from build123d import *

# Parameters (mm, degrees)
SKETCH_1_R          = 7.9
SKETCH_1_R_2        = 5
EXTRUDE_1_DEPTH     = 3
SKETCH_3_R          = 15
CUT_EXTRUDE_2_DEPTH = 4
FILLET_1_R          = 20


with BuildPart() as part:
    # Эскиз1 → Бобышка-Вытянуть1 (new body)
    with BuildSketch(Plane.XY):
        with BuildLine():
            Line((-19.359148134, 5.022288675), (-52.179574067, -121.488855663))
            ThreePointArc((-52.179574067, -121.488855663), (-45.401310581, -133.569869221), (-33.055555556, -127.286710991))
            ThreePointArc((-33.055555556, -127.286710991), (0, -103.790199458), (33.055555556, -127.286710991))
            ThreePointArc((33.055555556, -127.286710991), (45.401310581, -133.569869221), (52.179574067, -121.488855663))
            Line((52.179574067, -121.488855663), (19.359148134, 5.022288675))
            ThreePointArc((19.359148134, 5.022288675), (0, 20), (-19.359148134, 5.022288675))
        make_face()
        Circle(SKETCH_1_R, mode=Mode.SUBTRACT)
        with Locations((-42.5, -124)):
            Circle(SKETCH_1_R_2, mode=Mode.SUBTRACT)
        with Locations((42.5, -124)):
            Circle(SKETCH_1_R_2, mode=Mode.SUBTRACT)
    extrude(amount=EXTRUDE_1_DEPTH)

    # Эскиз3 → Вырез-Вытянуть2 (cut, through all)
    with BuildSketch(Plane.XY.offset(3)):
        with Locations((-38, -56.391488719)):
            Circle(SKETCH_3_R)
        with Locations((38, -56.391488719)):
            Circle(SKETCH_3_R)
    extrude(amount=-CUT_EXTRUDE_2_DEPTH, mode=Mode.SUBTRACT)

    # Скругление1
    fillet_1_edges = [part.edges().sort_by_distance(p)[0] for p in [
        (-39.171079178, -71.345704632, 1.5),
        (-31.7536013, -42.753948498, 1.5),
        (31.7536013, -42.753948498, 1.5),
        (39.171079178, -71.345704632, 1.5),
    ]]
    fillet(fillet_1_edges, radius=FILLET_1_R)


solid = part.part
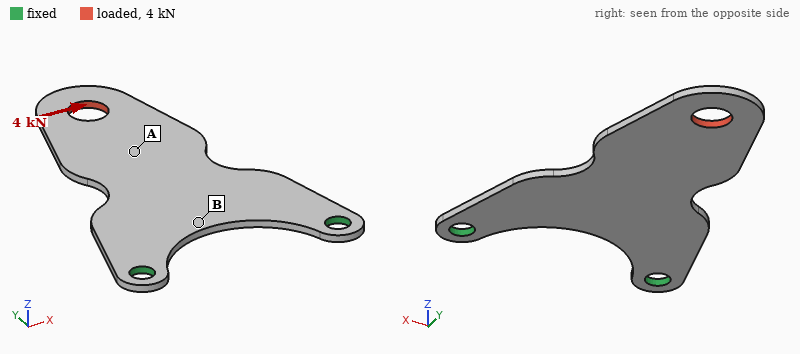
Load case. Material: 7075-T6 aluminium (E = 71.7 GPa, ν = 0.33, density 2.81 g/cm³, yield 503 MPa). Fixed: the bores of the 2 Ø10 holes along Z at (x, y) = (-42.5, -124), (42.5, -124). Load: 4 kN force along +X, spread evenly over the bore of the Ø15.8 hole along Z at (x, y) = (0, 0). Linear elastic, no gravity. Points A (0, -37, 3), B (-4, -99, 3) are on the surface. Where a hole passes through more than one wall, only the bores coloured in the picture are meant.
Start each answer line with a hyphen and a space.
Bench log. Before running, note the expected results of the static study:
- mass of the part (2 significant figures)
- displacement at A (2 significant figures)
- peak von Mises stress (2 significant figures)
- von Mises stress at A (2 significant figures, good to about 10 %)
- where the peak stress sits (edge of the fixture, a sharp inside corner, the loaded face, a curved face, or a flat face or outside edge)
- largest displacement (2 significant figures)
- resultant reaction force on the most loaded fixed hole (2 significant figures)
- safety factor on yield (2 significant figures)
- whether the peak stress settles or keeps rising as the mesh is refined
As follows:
- 69 g
- 0.23 mm
- 340 MPa
- 78 MPa
- a curved face
- 0.68 mm
- 6.1 kN
- 1.5
- settles
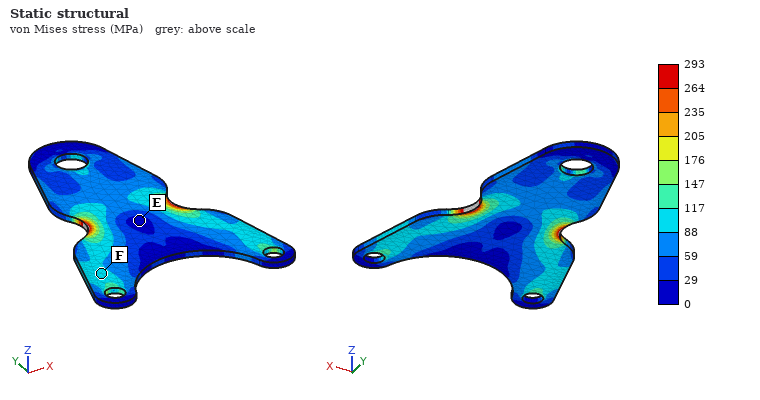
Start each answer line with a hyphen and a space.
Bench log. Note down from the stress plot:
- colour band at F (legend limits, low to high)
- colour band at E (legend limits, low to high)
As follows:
- 88 to 117 MPa
- 0 to 29 MPa
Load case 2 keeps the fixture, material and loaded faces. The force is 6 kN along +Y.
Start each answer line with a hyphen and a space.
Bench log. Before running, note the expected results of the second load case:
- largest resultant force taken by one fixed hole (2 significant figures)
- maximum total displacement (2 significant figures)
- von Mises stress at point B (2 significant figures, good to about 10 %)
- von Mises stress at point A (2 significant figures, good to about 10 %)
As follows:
- 3.3 kN
- 96 µm
- 9.2 MPa
- 43 MPa
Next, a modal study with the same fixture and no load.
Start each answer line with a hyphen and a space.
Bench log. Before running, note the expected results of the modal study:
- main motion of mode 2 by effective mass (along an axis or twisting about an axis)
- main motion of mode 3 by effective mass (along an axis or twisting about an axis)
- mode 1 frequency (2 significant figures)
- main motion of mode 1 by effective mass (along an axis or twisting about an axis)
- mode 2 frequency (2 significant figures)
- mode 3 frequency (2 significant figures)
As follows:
- along Z
- twisting about Y
- 150 Hz
- along Z
- 780 Hz
- 880 Hz
